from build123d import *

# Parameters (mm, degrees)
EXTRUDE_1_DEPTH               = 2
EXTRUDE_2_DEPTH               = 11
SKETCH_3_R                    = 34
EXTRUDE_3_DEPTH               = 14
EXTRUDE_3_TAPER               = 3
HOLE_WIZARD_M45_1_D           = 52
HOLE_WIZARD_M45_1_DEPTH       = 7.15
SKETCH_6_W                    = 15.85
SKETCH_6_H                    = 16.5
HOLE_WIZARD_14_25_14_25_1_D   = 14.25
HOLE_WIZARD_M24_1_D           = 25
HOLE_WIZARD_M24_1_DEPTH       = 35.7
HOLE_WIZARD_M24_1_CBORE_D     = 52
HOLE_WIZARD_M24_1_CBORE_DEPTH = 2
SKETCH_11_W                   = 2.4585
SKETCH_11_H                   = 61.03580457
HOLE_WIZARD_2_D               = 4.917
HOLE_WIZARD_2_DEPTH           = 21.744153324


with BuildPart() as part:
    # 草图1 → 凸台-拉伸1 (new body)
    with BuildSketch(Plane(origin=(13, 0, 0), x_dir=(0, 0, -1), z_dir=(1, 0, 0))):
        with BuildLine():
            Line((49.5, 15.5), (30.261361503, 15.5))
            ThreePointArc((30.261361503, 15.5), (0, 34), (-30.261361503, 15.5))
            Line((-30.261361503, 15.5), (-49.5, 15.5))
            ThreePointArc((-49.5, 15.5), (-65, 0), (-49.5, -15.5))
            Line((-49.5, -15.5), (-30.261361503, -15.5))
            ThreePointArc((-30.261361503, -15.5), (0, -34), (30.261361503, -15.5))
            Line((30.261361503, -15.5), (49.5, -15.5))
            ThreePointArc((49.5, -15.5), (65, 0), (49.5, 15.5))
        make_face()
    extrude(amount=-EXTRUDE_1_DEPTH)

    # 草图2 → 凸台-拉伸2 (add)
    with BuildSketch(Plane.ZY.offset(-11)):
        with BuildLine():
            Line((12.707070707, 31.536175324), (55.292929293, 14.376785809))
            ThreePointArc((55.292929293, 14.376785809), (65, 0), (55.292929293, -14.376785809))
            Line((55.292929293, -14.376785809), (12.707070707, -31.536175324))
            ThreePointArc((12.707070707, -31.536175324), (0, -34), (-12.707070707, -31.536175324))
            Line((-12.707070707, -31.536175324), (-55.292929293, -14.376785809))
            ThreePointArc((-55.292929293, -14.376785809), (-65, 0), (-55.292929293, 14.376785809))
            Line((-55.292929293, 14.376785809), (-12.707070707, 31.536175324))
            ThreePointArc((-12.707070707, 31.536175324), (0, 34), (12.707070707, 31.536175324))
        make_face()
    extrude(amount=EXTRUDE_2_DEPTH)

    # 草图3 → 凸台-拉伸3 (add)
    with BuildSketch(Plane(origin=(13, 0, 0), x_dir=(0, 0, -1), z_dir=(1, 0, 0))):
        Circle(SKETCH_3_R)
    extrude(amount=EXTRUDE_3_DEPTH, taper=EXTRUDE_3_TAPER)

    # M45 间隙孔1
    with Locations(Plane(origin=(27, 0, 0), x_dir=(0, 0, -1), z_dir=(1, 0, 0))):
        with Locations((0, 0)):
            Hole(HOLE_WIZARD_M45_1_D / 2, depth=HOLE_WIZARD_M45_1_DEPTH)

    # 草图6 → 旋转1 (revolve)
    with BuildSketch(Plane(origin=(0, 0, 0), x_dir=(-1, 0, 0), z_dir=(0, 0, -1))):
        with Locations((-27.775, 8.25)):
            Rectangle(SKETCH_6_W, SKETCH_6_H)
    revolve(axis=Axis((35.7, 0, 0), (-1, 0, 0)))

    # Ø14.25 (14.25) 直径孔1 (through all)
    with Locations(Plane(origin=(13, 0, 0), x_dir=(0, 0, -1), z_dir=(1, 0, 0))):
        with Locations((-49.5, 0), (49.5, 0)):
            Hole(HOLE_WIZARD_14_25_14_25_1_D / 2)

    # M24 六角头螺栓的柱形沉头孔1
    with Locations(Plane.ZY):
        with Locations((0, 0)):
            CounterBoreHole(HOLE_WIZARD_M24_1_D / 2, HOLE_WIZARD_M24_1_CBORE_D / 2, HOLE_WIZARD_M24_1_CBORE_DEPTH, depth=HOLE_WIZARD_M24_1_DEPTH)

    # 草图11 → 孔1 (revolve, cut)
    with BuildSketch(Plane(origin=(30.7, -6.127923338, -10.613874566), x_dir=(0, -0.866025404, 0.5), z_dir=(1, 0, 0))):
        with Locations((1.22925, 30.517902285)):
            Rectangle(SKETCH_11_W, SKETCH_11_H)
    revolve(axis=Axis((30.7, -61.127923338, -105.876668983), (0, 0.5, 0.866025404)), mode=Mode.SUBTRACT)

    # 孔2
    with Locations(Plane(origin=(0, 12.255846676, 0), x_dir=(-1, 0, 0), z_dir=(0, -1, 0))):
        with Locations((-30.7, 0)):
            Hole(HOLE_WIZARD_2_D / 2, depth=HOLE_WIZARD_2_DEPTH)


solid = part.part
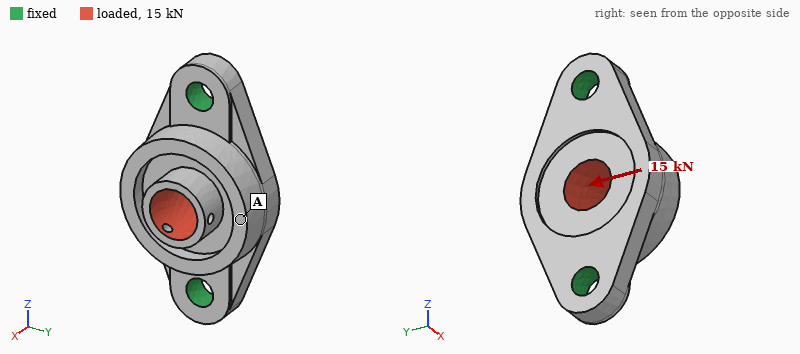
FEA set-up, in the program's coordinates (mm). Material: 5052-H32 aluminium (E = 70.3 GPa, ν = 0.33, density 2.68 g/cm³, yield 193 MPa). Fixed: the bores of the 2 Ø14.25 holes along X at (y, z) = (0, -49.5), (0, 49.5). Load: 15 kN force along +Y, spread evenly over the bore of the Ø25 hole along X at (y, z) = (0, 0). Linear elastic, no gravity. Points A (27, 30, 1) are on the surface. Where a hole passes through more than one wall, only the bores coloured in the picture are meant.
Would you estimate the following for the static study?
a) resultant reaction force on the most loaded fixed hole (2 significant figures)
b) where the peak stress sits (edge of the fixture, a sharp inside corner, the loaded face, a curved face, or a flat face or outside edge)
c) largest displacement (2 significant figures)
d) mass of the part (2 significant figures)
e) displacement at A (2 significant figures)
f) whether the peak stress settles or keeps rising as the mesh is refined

7.5 kN
edge of the fixture
0.12 mm
270 g
0.098 mm
keeps rising
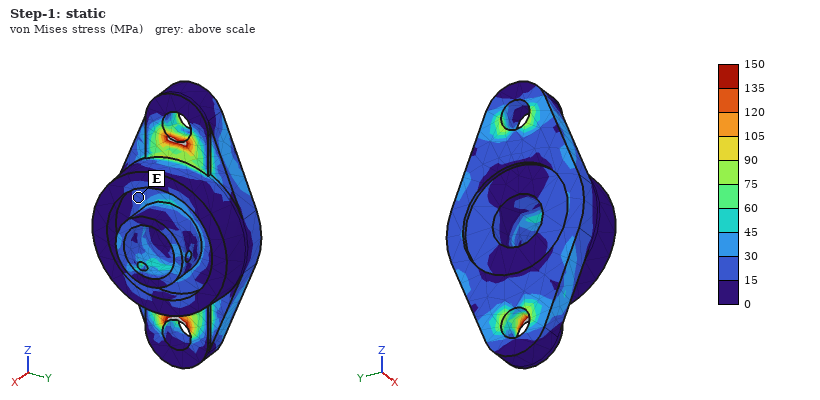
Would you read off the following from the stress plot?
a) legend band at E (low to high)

15 to 30 MPa
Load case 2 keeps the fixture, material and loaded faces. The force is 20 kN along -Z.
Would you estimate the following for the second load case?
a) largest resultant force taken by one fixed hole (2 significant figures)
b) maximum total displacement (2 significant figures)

10 kN
46 µm
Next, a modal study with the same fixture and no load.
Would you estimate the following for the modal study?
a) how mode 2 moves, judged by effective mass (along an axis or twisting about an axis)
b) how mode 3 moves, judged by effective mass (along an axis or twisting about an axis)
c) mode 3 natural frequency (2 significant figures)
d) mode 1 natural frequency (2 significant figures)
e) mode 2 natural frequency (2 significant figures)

along X
along Y
11 kHz
4600 Hz
6100 Hz
